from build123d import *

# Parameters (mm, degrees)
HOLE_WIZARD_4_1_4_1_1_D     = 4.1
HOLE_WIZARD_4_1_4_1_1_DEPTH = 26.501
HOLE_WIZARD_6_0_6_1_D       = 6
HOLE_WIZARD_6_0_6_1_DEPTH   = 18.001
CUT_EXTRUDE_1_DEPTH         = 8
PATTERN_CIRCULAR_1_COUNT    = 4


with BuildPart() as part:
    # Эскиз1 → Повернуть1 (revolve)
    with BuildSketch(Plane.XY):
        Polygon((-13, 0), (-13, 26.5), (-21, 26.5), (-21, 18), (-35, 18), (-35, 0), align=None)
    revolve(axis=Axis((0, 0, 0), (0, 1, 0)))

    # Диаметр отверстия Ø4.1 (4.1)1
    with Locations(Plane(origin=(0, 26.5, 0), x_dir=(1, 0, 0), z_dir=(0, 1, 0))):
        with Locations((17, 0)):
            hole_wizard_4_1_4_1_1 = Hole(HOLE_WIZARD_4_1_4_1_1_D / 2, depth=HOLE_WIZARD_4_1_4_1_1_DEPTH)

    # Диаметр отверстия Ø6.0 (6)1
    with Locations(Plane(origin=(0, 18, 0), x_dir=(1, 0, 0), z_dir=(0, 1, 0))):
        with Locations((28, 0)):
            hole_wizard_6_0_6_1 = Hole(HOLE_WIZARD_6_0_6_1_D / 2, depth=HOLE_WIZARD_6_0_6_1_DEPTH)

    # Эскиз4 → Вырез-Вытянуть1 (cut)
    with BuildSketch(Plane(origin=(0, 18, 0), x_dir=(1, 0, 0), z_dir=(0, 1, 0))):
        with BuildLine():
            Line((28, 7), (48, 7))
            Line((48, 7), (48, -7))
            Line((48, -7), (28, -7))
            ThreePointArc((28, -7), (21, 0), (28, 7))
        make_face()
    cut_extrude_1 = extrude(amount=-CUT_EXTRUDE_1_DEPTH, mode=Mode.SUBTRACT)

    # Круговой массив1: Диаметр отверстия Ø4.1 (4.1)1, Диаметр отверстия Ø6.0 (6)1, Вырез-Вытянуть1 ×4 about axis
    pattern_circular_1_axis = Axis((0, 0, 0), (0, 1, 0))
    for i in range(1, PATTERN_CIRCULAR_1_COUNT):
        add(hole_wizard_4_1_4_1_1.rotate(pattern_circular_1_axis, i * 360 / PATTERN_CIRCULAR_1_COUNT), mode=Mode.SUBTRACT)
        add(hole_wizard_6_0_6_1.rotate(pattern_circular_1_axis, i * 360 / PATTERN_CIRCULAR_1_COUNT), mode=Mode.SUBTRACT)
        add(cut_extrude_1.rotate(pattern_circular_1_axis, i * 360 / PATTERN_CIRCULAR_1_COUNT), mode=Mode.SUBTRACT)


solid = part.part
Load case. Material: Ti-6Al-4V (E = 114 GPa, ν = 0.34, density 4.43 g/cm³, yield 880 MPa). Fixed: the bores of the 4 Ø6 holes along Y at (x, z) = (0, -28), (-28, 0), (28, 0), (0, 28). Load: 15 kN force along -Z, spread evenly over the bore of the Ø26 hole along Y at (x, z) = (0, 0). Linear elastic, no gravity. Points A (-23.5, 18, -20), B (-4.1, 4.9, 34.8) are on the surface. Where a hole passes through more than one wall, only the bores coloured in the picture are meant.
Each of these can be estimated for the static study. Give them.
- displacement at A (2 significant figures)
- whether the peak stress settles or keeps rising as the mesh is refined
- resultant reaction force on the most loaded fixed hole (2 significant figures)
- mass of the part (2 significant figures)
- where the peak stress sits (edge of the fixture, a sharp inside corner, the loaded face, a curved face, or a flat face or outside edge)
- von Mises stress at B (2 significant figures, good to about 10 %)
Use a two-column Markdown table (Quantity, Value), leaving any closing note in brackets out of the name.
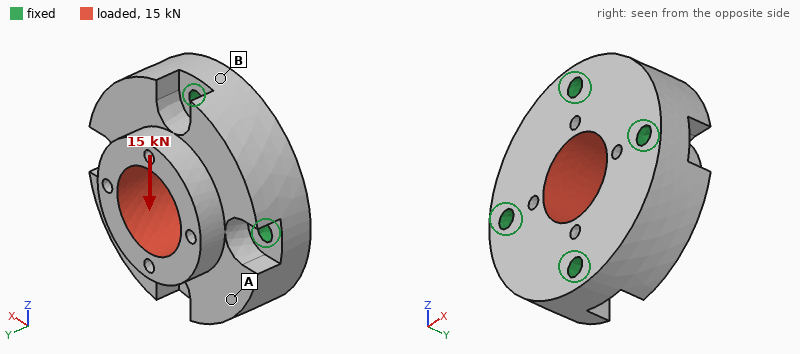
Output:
| Quantity | Value |
|---|---|
| displacement at A | 4.4 µm |
| whether the peak stress settles or keeps rising as the mesh is refined | keeps rising |
| resultant reaction force on the most loaded fixed hole | 4.7 kN |
| mass of the part | 260 g |
| where the peak stress sits | edge of the fixture |
| von Mises stress at B | 16 MPa |
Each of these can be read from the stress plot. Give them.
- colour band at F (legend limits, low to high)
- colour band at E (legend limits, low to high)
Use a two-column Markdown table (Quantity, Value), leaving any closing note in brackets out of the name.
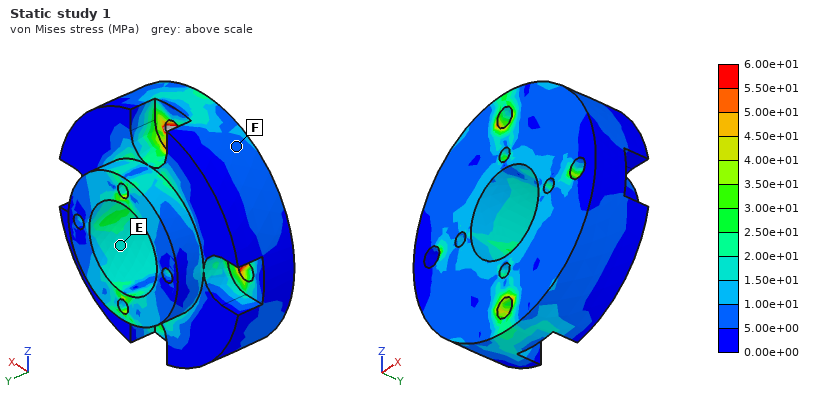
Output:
| Quantity | Value |
|---|---|
| colour band at F | 5.00e+00 to 1.00e+01 MPa |
| colour band at E | 1.50e+01 to 2.00e+01 MPa |
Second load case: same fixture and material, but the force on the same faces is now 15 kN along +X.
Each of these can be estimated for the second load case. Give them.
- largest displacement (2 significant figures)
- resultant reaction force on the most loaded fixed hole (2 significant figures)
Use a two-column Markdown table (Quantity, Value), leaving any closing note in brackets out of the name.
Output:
| Quantity | Value |
|---|---|
| largest displacement | 9.1 µm |
| resultant reaction force on the most loaded fixed hole | 4.7 kN |
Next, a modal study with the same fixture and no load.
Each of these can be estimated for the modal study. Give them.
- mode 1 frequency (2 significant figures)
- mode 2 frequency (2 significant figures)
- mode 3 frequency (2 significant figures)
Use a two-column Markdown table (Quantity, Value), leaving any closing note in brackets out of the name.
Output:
| Quantity | Value |
|---|---|
| mode 1 frequency | 17 kHz |
| mode 2 frequency | 19 kHz |
| mode 3 frequency | 19 kHz |
